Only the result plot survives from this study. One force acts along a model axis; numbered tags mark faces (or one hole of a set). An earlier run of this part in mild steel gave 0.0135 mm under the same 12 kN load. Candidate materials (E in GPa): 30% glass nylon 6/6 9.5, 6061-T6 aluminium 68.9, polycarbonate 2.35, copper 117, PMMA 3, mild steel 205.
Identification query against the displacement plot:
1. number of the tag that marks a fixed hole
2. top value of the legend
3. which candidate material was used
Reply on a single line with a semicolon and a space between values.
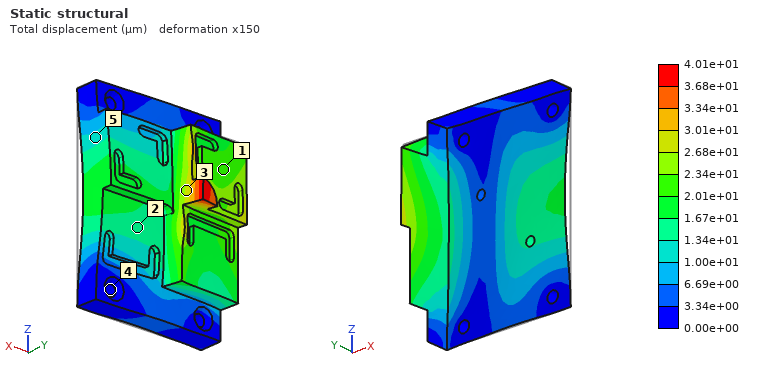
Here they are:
4; 4.01e+01 µm; 6061-T6 aluminium
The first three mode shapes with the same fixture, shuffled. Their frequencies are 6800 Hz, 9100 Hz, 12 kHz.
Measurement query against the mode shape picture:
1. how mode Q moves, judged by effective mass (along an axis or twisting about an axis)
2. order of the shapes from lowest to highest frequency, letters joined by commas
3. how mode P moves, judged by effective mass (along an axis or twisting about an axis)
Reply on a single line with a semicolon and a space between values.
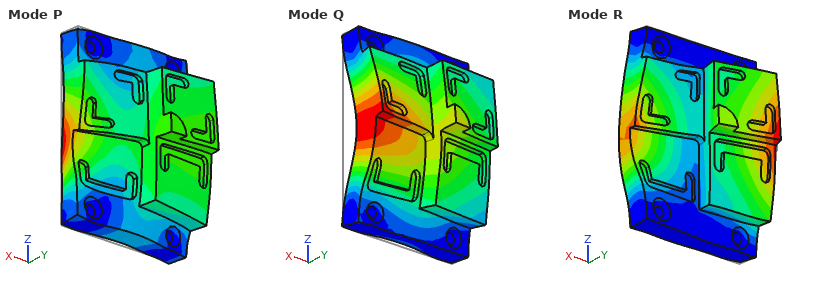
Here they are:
along Y; Q, R, P; along X
